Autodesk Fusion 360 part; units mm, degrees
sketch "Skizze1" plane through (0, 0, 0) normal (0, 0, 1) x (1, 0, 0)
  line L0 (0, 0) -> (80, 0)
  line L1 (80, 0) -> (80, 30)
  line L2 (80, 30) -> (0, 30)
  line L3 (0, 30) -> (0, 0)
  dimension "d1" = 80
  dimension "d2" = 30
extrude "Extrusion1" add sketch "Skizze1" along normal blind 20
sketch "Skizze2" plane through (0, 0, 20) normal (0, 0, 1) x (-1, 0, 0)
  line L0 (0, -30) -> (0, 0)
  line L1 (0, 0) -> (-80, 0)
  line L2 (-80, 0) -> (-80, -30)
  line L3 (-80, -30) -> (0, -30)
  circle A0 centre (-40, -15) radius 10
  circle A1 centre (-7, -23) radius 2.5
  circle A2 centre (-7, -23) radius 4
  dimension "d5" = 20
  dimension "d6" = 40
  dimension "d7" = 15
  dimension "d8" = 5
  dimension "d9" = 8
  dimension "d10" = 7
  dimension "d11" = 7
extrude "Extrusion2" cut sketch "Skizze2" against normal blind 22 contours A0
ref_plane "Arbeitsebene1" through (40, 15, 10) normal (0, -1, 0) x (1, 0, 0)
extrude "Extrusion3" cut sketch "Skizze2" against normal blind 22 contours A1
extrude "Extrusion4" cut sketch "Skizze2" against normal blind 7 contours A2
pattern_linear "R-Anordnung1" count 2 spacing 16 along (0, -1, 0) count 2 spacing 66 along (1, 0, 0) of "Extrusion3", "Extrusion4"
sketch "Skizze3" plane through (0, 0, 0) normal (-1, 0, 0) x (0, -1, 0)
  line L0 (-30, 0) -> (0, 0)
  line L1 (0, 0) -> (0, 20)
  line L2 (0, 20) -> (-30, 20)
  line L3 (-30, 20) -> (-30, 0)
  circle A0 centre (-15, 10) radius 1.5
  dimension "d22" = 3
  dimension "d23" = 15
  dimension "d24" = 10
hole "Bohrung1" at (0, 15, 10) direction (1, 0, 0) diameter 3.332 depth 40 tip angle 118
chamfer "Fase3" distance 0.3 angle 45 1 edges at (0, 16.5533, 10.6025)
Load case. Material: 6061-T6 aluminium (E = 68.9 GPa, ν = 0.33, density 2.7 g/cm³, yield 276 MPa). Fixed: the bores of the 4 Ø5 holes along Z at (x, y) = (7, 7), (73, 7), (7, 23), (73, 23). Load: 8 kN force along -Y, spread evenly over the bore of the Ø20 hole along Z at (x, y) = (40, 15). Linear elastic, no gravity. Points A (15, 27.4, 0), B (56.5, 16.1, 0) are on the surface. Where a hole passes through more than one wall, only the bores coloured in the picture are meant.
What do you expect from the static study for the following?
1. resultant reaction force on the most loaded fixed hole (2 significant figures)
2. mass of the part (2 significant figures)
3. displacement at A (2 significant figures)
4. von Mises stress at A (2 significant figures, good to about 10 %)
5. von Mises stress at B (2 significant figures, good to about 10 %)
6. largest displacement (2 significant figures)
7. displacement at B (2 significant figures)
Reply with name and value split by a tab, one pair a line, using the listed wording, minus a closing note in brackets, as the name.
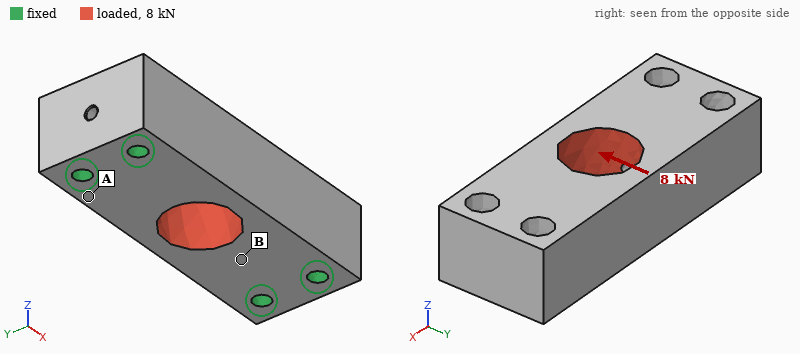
resultant reaction force on the most loaded fixed hole	3.4 kN
mass of the part	110 g
displacement at A	4.2 µm
von Mises stress at A	7.8 MPa
von Mises stress at B	23 MPa
largest displacement	17 µm
displacement at B	8.0 µm
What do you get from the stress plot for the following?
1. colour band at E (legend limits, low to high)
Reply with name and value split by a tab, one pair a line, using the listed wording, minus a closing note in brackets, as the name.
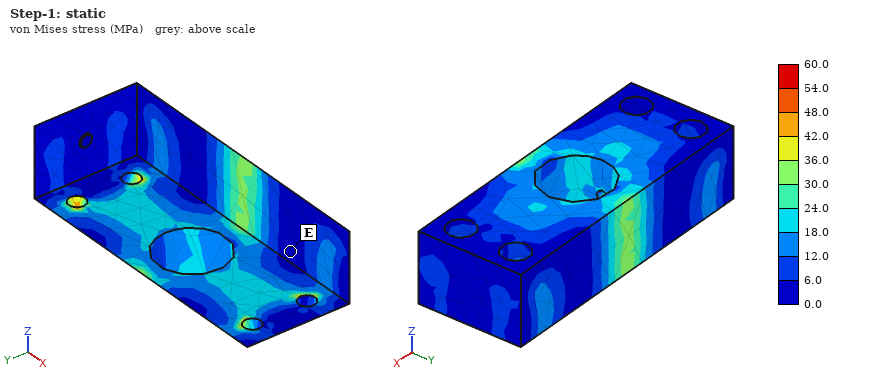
colour band at E	0.0 to 6.0 MPa
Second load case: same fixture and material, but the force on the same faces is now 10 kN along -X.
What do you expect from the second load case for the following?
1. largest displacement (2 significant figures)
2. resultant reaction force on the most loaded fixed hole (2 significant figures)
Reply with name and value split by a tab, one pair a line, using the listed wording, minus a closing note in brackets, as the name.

largest displacement	4.9 µm
resultant reaction force on the most loaded fixed hole	2.5 kN
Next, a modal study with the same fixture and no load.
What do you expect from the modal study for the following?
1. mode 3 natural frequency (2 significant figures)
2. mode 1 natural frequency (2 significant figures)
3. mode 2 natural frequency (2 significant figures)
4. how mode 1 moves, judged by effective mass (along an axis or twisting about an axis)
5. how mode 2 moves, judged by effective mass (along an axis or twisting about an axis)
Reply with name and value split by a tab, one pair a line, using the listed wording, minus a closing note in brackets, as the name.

mode 3 natural frequency	21 kHz
mode 1 natural frequency	14 kHz
mode 2 natural frequency	19 kHz
how mode 1 moves, judged by effective mass	along Z
how mode 2 moves, judged by effective mass	along Y
